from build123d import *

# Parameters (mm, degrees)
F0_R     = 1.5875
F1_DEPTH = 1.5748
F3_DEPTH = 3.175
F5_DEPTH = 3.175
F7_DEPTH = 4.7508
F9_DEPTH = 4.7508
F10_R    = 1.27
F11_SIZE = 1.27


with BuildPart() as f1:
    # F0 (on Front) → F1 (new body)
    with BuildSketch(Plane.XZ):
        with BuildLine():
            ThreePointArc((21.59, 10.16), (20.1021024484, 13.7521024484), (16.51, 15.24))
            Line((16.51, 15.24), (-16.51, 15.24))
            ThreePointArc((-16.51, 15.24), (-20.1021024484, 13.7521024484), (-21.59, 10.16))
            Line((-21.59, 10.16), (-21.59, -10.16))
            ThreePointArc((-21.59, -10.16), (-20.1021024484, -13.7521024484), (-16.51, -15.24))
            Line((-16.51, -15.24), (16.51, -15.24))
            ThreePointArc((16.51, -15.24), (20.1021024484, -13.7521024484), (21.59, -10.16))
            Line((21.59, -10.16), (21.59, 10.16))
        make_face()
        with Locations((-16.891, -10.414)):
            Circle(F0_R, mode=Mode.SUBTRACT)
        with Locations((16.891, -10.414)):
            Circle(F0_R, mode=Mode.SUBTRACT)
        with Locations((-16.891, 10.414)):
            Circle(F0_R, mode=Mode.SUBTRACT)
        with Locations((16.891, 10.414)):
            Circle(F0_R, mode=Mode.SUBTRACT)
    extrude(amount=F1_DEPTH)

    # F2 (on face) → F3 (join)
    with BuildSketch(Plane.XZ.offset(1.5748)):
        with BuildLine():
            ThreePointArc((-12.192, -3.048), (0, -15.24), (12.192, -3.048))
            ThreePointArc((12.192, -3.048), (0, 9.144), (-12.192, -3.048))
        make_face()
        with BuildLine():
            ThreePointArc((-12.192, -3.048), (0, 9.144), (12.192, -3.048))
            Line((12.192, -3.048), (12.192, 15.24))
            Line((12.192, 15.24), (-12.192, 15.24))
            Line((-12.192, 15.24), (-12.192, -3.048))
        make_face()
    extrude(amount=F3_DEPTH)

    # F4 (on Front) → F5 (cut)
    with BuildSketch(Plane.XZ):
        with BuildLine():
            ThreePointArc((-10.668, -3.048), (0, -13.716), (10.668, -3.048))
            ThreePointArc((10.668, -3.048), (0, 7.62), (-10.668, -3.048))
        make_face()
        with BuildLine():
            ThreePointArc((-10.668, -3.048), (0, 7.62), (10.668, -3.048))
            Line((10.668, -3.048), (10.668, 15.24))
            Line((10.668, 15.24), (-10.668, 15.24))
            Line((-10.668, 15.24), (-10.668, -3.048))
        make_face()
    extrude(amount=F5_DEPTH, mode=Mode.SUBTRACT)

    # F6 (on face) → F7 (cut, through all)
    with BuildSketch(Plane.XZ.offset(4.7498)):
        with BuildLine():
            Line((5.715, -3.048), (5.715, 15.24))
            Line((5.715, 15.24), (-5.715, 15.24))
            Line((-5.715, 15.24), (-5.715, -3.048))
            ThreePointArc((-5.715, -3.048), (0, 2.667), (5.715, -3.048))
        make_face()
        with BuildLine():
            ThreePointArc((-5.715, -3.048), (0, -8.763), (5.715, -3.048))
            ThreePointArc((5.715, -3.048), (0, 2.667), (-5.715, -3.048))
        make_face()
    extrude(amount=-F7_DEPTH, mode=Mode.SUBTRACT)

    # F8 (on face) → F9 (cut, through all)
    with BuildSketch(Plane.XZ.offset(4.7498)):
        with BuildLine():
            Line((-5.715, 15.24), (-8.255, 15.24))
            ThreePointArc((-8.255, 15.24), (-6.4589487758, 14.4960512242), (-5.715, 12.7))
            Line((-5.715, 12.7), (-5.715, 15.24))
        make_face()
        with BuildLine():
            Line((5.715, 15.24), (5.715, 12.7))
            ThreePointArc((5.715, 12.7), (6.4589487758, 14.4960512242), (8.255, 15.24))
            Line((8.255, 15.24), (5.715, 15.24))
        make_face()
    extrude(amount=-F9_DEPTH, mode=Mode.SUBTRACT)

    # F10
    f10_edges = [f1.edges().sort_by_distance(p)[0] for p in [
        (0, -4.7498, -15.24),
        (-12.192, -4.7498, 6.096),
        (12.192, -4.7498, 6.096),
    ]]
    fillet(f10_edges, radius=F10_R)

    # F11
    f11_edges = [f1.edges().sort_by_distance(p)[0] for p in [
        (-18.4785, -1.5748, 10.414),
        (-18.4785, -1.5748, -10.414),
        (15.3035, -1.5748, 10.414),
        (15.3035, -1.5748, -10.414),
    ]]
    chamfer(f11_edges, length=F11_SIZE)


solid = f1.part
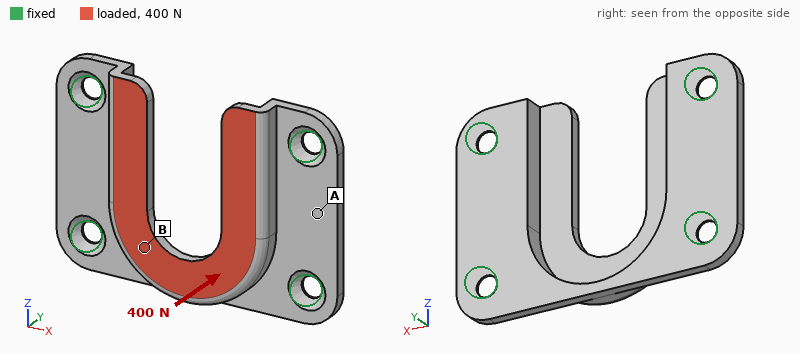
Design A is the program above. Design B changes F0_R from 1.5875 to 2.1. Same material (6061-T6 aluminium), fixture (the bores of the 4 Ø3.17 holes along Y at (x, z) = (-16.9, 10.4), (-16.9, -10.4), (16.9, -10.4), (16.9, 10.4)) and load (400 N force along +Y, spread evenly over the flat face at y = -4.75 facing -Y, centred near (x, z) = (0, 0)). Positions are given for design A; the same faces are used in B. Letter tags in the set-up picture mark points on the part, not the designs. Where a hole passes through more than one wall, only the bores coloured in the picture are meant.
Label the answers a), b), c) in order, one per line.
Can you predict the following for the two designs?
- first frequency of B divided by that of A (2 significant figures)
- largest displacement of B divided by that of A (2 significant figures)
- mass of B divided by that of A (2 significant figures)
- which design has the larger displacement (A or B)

a) 1.1
b) 0.84
c) 0.97
d) A
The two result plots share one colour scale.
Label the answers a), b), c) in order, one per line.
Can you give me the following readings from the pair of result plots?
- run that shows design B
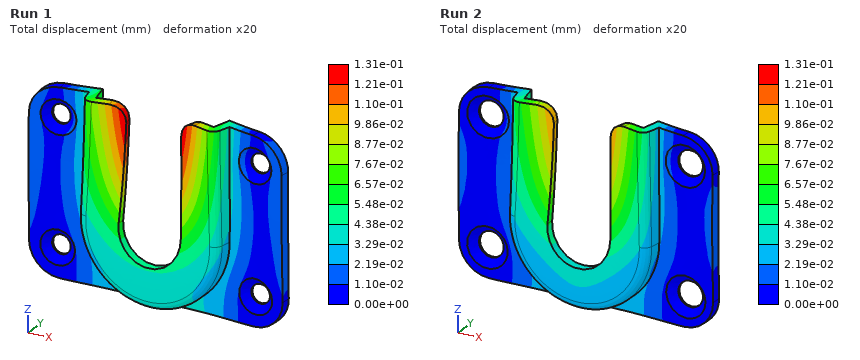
a) Run 2
